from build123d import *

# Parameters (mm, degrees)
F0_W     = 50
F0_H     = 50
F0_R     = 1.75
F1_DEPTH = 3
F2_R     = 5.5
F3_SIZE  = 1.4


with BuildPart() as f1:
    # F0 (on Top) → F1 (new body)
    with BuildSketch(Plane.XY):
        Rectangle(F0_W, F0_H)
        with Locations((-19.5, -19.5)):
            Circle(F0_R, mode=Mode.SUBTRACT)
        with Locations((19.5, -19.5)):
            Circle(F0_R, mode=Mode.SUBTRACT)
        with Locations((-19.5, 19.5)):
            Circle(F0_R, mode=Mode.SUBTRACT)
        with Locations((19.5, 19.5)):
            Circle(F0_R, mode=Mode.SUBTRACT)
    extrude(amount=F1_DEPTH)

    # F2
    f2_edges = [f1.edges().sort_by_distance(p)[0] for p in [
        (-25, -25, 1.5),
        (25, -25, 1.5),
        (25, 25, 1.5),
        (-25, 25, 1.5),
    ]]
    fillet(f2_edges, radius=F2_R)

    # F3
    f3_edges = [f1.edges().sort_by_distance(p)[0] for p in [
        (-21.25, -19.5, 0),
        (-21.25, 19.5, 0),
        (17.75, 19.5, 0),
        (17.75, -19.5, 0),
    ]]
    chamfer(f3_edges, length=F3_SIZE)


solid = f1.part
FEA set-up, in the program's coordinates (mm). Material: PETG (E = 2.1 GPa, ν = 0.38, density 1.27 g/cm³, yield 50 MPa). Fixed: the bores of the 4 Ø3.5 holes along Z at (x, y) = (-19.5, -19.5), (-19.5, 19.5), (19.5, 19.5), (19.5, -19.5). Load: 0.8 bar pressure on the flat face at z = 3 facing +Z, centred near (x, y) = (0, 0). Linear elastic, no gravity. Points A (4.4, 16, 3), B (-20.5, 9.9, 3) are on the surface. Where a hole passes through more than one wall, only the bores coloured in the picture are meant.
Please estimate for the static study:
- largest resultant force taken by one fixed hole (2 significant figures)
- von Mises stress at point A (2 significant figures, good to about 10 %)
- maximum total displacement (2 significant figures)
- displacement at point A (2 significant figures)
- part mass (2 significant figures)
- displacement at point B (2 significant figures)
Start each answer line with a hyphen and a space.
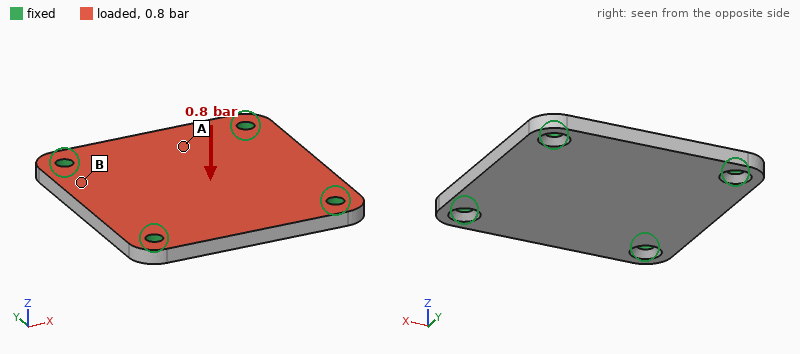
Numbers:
- 61 N
- 3.5 MPa
- 0.30 mm
- 0.19 mm
- 9.2 g
- 0.10 mm
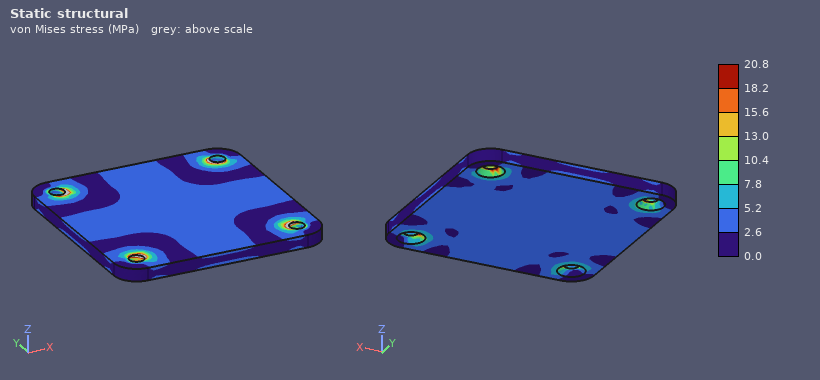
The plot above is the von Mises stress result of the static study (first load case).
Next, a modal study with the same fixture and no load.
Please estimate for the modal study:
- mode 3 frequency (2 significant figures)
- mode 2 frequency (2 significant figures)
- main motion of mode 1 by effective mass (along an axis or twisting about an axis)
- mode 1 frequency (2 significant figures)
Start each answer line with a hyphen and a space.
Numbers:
- 2600 Hz
- 2500 Hz
- along Z
- 1600 Hz
